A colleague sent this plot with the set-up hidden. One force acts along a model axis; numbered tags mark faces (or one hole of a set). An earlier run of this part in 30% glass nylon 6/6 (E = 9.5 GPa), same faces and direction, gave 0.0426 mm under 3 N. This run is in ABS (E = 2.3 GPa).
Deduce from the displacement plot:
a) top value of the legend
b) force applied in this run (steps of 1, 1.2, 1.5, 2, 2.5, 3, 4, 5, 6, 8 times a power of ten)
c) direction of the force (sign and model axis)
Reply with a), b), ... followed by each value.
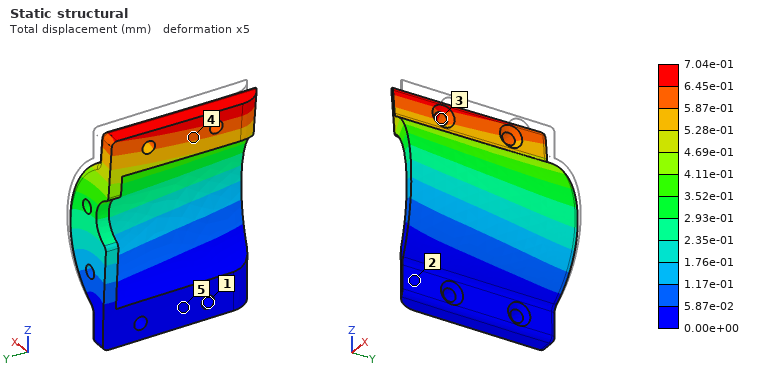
a) 7.04e-01 mm
b) 12 N
c) -X
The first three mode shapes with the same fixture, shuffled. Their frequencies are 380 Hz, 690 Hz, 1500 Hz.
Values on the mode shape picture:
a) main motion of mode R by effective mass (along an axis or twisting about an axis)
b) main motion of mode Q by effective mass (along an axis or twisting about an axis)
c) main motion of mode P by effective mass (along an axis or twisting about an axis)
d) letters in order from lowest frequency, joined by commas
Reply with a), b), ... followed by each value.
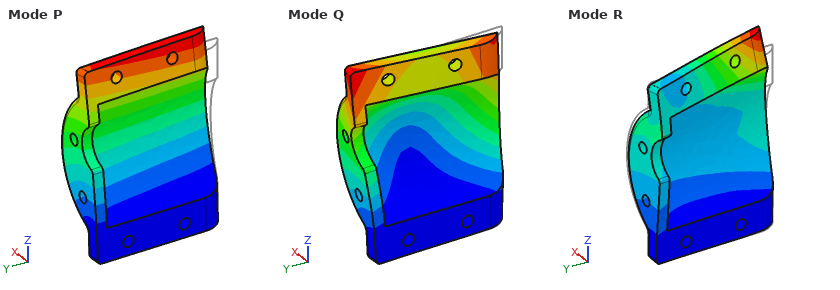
a) along Z
b) along Y
c) along X
d) P, Q, R
